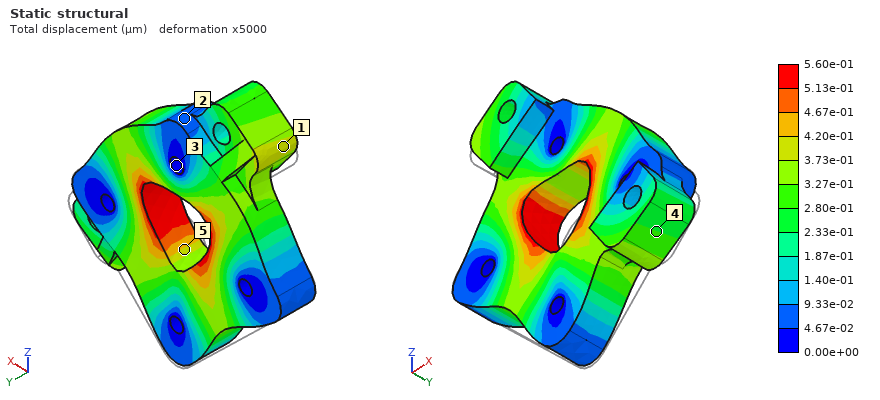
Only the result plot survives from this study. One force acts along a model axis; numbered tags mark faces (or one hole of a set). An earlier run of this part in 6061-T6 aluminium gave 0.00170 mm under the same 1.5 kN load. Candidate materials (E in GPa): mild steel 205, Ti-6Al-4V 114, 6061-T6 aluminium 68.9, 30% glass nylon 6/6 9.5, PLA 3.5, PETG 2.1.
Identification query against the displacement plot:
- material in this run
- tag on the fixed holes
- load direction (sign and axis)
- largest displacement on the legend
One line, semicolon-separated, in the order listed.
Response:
mild steel; 3; +Z; 5.60e-01 µm
